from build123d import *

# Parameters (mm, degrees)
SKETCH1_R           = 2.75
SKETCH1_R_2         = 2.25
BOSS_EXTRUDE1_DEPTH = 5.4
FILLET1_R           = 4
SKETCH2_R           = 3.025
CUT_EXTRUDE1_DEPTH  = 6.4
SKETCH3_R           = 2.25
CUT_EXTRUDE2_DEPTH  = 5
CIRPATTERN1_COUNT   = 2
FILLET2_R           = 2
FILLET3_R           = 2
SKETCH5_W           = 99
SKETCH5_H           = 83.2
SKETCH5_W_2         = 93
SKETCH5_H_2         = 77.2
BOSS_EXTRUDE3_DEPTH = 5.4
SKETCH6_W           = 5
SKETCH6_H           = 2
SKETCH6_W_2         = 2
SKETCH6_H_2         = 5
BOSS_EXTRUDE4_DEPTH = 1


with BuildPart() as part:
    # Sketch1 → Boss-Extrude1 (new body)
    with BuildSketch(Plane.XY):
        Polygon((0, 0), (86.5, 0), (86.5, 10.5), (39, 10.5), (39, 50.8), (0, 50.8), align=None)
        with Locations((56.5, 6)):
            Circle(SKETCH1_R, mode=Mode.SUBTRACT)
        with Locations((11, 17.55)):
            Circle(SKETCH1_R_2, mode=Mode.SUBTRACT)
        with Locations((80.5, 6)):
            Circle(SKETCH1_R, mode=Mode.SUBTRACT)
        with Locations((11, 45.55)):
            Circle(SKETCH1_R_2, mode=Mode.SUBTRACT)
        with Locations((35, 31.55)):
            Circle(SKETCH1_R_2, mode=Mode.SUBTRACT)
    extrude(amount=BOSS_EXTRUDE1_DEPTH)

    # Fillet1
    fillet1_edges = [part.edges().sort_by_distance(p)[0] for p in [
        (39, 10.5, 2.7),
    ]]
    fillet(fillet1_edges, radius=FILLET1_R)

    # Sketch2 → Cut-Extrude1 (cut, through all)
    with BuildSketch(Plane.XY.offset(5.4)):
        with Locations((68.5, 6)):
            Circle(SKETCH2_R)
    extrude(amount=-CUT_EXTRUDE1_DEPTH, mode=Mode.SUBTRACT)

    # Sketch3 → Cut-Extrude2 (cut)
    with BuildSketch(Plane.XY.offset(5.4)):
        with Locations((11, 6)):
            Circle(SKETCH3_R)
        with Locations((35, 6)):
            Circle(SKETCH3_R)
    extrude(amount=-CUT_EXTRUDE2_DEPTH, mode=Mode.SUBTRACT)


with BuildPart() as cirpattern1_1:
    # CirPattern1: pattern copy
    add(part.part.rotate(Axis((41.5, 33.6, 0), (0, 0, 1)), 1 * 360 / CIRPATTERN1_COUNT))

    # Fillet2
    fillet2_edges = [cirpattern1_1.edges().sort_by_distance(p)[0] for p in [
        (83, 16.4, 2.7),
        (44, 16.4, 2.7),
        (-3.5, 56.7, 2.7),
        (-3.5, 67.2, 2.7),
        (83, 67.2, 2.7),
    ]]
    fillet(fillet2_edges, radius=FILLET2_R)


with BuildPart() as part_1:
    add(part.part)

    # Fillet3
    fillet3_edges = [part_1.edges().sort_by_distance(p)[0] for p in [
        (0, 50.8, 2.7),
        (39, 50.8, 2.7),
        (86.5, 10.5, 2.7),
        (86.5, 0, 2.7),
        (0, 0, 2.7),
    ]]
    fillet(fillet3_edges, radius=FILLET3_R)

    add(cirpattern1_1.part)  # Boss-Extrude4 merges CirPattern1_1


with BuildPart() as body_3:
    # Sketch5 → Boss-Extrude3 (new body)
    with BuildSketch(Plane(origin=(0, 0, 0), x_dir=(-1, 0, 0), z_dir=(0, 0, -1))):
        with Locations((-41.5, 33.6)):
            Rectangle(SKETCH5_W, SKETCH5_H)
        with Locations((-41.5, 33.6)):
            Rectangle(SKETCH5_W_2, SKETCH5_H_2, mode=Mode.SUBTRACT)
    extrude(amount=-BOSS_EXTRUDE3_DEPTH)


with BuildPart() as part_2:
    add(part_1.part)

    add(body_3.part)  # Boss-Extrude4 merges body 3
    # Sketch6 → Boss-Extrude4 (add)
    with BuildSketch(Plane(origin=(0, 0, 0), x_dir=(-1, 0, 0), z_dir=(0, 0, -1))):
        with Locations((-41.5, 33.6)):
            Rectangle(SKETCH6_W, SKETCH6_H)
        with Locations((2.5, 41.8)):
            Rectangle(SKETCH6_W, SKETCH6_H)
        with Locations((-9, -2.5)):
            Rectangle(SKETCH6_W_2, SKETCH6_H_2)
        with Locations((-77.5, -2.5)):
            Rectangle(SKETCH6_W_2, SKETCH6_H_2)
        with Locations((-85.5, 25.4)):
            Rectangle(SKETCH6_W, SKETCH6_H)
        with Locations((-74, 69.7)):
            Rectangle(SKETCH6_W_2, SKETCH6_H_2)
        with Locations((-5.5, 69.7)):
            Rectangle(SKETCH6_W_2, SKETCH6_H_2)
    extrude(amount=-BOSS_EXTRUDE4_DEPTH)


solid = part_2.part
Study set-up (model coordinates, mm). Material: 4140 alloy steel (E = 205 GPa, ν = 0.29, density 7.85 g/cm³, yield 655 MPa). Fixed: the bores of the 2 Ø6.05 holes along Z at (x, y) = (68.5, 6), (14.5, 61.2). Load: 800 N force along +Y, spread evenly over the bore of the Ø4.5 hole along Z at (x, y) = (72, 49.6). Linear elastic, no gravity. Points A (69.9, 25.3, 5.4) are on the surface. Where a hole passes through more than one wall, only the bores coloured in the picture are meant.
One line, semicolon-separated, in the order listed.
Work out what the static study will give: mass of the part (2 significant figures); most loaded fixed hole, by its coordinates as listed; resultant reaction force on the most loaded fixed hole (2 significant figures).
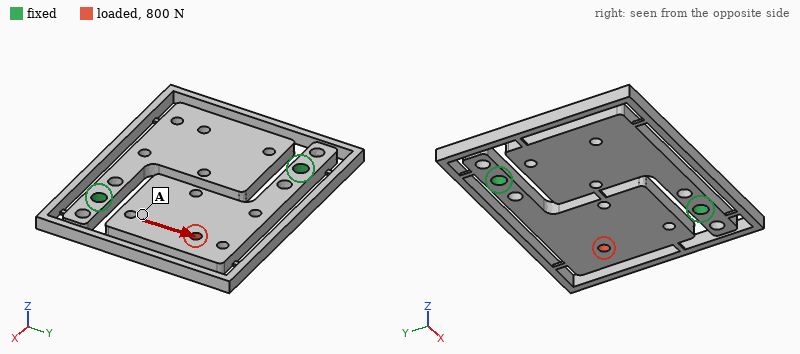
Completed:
240 g; (14.5, 61.2); 730 N
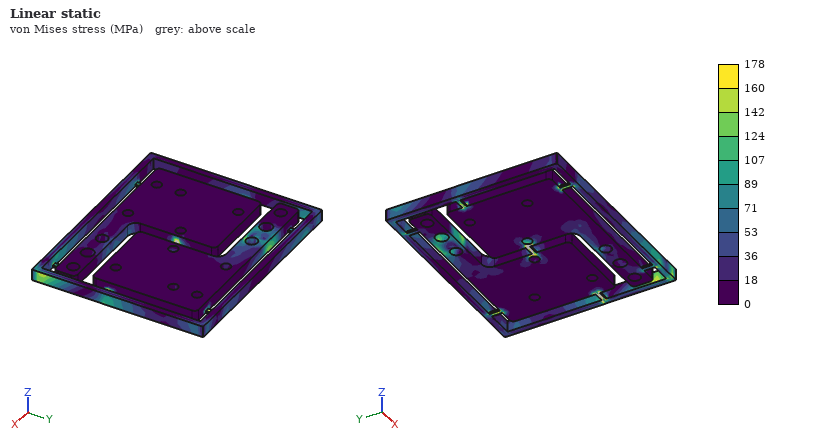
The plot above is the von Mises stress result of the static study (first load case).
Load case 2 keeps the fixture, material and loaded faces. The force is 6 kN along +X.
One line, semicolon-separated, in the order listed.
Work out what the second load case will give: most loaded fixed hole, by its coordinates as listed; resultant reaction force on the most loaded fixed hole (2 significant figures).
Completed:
(14.5, 61.2); 4.8 kN
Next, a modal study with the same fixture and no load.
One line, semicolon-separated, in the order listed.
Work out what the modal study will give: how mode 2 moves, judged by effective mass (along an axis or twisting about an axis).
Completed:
along Z
